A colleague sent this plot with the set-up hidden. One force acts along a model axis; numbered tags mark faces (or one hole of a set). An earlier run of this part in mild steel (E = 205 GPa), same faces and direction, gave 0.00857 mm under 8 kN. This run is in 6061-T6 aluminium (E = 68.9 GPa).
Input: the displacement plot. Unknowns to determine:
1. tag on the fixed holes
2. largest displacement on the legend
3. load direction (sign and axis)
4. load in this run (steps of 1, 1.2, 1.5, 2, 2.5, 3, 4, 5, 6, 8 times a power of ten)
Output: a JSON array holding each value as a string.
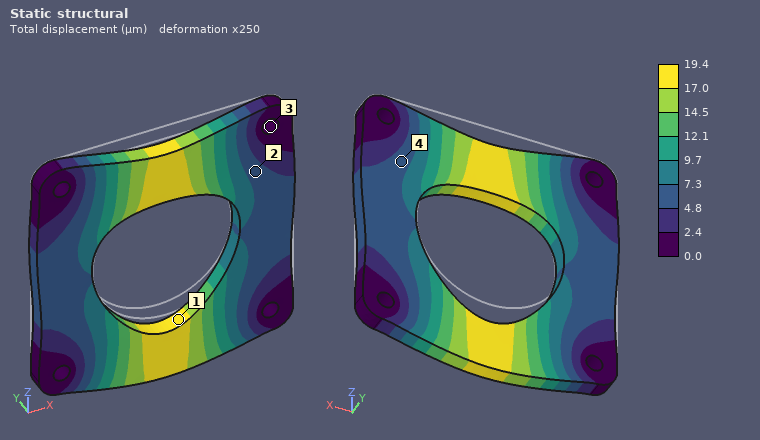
["3", "19.4 µm", "-Z", "6 kN"]
